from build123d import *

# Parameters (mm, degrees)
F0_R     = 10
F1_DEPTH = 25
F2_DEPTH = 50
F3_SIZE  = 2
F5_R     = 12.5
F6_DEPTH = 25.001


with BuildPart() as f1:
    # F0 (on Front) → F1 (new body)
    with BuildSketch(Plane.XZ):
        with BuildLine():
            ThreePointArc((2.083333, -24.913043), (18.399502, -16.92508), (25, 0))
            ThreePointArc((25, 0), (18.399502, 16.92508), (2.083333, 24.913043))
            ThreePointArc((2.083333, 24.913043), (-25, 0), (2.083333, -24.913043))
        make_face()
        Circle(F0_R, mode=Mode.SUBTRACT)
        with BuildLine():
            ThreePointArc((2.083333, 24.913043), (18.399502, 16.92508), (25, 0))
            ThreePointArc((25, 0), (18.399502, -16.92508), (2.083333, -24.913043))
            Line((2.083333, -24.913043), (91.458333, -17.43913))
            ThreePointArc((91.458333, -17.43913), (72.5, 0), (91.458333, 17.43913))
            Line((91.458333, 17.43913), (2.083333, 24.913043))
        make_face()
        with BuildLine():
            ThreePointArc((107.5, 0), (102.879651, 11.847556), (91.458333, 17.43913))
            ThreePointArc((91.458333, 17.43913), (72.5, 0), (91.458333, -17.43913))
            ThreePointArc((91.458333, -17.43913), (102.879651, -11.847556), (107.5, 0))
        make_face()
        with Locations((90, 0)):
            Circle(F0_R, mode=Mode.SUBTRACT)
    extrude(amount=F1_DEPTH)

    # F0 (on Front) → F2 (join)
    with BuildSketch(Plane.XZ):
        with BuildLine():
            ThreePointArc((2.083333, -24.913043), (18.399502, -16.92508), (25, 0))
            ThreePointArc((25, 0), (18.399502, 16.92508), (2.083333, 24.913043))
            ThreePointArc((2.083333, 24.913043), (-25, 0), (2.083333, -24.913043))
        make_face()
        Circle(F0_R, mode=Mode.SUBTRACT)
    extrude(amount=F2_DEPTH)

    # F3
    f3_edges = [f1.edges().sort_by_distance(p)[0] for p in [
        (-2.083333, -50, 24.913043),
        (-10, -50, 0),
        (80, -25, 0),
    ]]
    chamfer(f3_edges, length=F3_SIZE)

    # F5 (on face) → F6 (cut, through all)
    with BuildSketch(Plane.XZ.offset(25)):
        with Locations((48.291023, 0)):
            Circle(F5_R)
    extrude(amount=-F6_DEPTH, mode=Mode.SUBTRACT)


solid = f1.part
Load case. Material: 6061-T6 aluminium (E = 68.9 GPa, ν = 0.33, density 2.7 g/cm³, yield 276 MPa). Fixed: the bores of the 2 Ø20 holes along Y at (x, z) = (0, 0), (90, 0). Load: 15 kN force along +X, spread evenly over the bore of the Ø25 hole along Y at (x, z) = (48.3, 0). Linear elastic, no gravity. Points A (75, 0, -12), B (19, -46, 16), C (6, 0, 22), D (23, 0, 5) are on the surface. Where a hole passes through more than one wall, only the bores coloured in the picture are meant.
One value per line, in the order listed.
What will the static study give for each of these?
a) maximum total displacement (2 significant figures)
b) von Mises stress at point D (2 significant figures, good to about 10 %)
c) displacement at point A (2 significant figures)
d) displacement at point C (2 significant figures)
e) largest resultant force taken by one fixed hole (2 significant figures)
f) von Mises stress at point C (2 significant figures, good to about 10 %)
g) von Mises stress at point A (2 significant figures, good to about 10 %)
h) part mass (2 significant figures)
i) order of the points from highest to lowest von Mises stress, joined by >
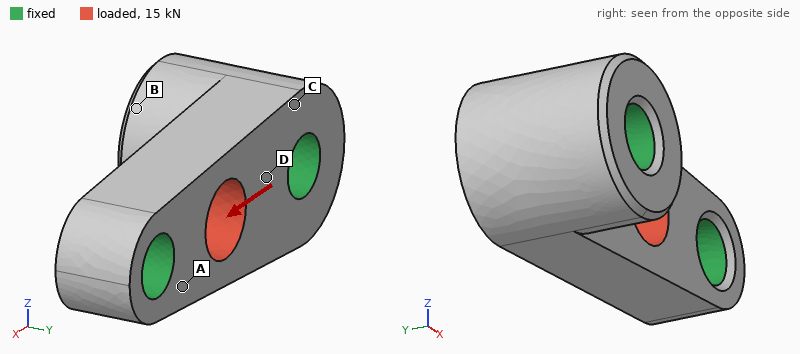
4.6 µm
9.0 MPa
1.5 µm
1.4 µm
7.7 kN
3.2 MPa
6.3 MPa
390 g
D > A > C > B
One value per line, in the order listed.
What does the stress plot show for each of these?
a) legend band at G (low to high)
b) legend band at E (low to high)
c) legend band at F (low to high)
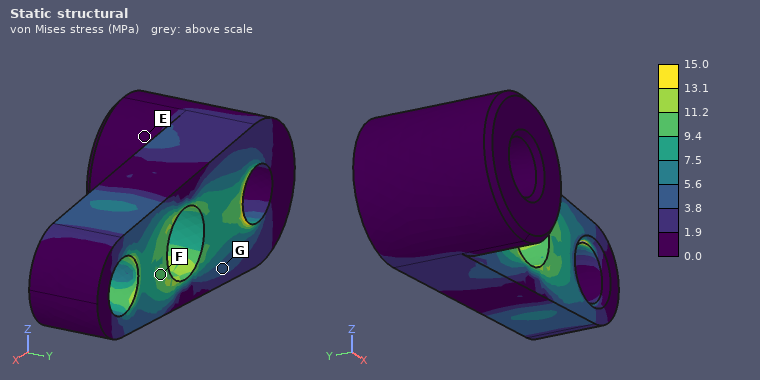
3.8 to 5.6 MPa
0.0 to 1.9 MPa
9.4 to 11.2 MPa
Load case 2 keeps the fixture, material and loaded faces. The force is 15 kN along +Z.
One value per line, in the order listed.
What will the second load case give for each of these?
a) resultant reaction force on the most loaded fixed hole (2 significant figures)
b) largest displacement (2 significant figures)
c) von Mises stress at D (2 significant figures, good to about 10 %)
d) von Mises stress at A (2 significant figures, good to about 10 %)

7.6 kN
17 µm
16 MPa
13 MPa
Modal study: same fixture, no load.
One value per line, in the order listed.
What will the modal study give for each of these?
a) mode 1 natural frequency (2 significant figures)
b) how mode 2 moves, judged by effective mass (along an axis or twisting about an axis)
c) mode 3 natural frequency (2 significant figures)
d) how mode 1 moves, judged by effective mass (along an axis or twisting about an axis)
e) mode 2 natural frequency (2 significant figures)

17 kHz
along Z
19 kHz
along Y
18 kHz
